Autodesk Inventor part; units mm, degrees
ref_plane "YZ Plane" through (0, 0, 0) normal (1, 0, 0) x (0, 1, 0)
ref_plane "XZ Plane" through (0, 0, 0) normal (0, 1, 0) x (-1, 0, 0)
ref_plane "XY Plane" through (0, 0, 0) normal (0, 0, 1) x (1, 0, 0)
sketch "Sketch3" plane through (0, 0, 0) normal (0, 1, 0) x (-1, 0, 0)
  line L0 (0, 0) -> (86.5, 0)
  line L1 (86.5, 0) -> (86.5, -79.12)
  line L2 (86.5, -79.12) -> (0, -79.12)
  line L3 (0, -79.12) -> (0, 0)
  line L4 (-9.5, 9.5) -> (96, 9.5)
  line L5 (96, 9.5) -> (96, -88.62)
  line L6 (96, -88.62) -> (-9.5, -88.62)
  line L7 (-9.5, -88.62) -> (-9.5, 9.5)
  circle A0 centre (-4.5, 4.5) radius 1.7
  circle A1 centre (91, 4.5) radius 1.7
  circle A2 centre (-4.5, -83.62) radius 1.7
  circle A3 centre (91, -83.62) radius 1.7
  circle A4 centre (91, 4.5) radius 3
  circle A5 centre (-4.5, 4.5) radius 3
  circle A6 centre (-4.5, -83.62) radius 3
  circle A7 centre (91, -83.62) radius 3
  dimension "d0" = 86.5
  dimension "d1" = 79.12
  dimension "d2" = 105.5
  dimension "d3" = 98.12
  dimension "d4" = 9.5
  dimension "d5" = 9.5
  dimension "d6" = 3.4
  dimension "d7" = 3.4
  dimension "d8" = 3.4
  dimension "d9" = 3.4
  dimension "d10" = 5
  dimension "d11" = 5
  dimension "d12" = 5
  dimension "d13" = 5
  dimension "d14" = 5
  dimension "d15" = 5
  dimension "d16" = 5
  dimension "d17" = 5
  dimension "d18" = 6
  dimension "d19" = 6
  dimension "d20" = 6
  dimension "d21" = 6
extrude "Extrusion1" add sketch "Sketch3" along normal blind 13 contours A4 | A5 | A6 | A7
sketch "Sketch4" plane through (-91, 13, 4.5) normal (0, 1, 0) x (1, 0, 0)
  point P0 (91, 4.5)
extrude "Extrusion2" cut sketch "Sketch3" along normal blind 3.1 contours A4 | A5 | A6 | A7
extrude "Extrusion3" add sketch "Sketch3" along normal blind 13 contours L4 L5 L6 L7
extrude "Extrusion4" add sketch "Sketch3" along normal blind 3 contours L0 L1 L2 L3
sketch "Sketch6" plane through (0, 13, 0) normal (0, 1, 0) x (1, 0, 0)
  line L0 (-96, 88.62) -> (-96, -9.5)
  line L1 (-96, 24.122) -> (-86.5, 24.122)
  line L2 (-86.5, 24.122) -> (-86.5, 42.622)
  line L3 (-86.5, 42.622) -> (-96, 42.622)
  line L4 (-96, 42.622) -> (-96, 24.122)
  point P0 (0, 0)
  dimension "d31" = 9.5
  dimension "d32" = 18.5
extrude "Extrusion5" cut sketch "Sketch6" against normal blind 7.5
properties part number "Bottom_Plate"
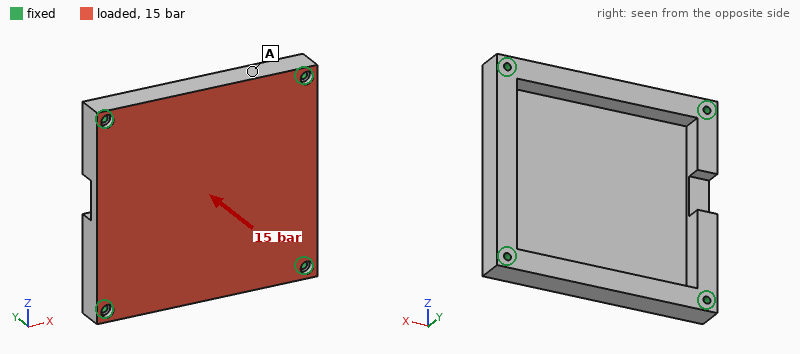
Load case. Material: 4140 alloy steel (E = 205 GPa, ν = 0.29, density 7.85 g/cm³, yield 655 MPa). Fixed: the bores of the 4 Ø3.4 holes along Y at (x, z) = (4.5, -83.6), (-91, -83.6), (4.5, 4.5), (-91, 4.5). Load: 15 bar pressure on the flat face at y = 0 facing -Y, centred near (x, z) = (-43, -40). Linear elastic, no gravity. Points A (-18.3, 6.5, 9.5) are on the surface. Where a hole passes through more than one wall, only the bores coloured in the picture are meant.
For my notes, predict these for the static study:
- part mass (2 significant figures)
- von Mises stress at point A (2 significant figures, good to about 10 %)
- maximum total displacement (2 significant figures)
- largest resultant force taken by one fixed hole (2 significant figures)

500 g
44 MPa
0.30 mm
6.5 kN
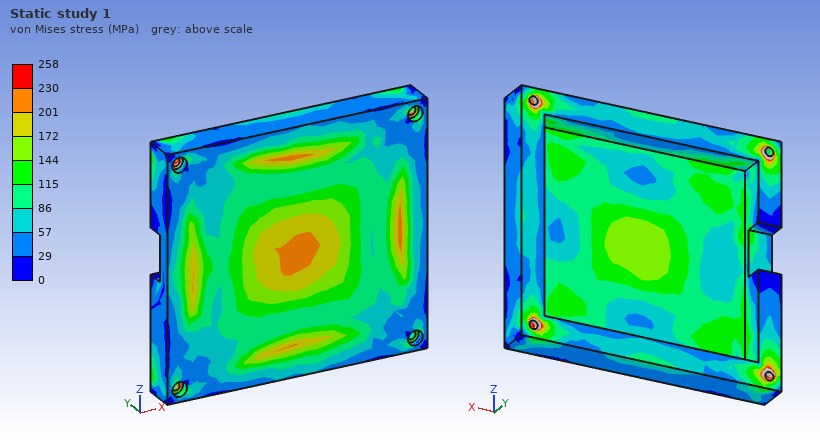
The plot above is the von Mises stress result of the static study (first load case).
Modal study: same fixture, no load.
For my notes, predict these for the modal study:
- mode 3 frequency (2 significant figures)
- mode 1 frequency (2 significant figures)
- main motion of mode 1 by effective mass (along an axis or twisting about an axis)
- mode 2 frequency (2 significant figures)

5300 Hz
3000 Hz
along Y
5100 Hz
